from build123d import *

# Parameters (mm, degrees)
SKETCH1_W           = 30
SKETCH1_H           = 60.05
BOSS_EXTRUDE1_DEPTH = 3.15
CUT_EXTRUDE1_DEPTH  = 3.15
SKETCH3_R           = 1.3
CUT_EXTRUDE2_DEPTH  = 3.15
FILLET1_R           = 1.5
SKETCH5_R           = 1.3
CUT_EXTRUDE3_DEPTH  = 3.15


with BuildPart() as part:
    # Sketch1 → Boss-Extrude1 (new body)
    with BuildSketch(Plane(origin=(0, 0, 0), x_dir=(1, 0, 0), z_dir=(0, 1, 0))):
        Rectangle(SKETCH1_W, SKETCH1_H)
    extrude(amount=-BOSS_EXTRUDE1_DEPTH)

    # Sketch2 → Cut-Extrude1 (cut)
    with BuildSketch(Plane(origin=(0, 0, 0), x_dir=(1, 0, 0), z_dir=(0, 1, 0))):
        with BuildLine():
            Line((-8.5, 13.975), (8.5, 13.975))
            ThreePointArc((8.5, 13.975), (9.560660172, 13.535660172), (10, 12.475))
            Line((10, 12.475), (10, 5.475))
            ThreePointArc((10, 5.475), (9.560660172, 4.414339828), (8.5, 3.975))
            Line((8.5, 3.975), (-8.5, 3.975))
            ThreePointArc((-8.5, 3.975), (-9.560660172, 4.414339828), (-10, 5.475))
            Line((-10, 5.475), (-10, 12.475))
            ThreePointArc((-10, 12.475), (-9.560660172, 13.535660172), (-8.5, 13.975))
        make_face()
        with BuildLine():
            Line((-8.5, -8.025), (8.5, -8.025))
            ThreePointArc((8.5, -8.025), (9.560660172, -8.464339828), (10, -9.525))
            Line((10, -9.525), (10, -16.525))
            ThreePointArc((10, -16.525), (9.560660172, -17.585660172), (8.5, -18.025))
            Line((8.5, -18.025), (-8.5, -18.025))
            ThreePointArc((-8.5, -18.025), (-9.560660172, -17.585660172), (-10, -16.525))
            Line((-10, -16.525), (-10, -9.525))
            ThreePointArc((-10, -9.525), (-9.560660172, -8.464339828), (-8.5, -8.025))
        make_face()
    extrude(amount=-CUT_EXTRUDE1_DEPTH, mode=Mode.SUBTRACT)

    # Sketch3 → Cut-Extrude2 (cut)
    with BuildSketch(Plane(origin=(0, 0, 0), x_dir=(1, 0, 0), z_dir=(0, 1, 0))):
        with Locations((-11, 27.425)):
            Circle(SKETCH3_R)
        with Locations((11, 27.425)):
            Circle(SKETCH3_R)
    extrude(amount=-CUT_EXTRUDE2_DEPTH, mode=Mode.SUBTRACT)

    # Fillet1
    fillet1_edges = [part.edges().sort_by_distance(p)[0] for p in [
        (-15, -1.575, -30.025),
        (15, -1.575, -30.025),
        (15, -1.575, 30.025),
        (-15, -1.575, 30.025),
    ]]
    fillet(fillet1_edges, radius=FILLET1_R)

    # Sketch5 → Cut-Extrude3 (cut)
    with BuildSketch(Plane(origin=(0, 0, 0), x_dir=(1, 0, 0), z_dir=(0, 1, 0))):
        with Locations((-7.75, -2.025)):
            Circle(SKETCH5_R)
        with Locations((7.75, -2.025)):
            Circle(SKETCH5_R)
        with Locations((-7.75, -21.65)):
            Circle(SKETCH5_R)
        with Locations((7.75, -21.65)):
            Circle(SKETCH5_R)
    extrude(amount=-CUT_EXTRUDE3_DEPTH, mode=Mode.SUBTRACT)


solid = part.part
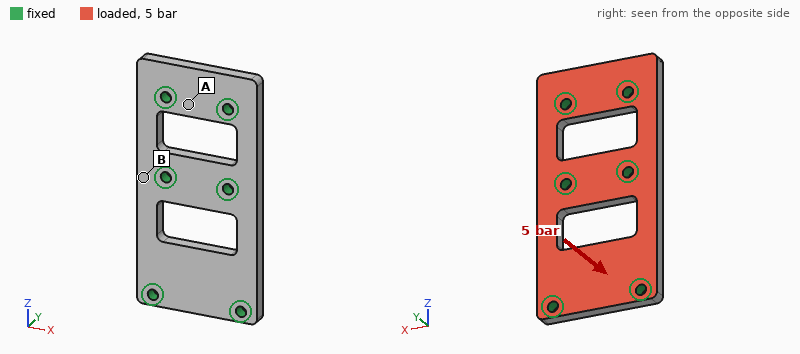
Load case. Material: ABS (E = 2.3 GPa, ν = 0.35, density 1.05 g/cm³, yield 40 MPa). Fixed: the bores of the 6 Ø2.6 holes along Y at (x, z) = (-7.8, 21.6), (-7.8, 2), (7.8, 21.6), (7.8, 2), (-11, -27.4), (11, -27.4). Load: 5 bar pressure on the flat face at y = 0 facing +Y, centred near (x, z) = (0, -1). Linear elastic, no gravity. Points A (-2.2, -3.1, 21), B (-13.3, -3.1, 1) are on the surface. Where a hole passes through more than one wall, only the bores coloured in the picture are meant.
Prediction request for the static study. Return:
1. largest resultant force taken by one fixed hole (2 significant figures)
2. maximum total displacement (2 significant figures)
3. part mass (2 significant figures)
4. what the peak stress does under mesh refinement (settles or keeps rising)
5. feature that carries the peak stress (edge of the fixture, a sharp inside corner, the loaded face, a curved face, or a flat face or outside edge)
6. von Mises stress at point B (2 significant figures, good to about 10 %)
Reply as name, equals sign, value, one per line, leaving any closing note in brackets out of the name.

largest resultant force taken by one fixed hole = 130 N
maximum total displacement = 0.35 mm
part mass = 4.5 g
what the peak stress does under mesh refinement = keeps rising
feature that carries the peak stress = edge of the fixture
von Mises stress at point B = 8.5 MPa
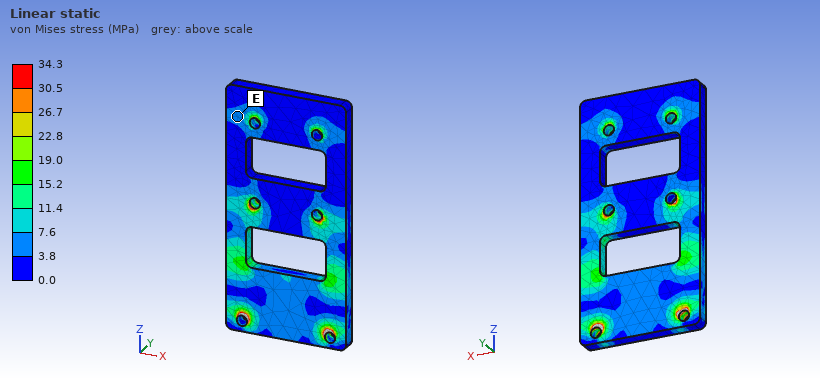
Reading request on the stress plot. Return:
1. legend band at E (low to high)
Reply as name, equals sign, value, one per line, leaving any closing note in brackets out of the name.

legend band at E = 3.8 to 7.6 MPa
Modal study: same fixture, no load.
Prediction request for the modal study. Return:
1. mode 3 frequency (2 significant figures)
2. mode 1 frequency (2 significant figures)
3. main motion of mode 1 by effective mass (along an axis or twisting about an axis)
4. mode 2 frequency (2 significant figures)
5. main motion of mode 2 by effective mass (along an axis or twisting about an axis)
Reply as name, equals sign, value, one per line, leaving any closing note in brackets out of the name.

mode 3 frequency = 7200 Hz
mode 1 frequency = 4400 Hz
main motion of mode 1 by effective mass = along Y
mode 2 frequency = 5800 Hz
main motion of mode 2 by effective mass = twisting about Z
